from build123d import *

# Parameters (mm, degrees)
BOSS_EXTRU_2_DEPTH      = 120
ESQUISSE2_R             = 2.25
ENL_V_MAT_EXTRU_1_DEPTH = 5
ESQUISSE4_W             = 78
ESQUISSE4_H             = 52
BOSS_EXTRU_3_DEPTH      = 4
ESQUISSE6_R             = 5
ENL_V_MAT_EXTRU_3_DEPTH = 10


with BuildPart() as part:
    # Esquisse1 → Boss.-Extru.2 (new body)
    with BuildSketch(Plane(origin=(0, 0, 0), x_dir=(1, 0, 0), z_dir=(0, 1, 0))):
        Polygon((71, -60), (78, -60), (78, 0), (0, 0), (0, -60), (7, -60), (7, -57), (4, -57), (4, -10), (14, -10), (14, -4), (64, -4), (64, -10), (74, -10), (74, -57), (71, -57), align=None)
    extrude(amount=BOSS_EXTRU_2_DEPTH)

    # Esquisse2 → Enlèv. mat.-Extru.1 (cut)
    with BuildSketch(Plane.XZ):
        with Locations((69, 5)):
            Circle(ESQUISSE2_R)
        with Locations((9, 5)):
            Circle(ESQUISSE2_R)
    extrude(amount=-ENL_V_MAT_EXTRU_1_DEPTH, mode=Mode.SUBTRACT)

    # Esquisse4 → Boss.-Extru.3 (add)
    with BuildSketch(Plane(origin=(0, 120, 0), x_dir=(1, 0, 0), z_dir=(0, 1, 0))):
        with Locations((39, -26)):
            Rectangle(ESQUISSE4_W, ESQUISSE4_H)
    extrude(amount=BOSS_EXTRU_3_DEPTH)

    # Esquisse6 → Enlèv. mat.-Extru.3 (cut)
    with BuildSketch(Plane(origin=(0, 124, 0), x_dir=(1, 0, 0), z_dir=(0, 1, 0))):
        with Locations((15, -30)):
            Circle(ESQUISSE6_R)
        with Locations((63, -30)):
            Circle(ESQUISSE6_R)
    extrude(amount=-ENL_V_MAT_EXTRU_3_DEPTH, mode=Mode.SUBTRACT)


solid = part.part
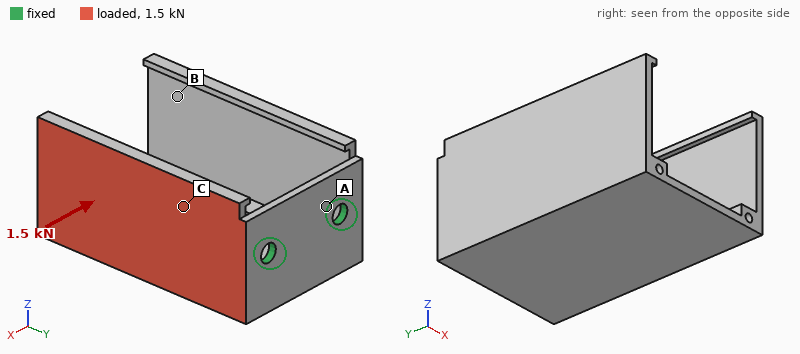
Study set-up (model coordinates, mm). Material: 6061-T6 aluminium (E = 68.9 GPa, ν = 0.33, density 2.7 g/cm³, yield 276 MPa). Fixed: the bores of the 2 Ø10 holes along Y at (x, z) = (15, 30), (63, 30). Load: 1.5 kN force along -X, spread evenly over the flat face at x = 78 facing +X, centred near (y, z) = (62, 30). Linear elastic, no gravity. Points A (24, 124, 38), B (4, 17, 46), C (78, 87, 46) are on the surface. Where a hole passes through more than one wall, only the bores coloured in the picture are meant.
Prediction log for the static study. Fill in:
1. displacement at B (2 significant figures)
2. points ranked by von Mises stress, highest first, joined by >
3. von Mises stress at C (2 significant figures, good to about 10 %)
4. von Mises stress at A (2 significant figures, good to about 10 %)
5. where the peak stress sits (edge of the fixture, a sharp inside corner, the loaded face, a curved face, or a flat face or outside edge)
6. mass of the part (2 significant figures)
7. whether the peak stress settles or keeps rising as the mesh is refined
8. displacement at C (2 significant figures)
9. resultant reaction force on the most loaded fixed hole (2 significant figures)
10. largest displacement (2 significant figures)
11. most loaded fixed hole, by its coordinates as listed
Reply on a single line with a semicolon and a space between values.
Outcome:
0.77 mm; C > A > B; 45 MPa; 27 MPa; edge of the fixture; 330 g; keeps rising; 0.49 mm; 1.6 kN; 1.8 mm; (63, 30)
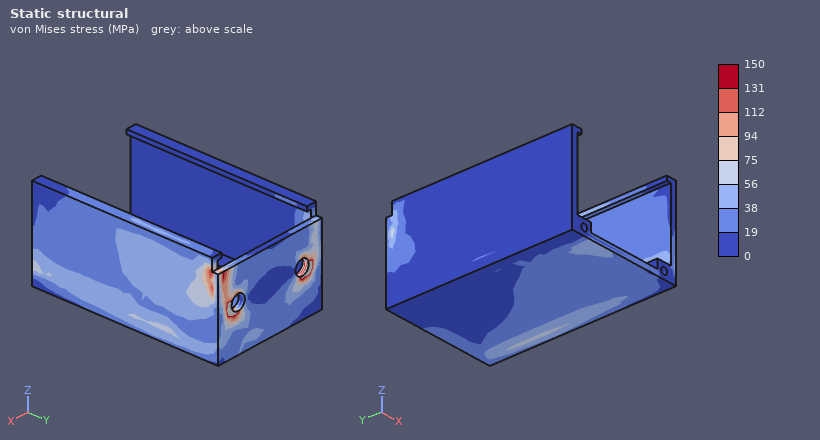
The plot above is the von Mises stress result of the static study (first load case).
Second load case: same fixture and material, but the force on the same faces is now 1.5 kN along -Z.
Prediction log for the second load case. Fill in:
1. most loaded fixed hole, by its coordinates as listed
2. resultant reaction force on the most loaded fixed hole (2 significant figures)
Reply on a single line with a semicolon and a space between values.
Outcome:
(63, 30); 1.8 kN
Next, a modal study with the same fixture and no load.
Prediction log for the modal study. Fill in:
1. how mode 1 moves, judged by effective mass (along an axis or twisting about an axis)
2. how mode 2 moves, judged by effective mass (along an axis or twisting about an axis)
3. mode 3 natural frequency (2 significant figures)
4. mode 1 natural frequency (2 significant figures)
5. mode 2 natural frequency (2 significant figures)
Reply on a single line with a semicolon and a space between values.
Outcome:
along Z; along X; 910 Hz; 380 Hz; 450 Hz
